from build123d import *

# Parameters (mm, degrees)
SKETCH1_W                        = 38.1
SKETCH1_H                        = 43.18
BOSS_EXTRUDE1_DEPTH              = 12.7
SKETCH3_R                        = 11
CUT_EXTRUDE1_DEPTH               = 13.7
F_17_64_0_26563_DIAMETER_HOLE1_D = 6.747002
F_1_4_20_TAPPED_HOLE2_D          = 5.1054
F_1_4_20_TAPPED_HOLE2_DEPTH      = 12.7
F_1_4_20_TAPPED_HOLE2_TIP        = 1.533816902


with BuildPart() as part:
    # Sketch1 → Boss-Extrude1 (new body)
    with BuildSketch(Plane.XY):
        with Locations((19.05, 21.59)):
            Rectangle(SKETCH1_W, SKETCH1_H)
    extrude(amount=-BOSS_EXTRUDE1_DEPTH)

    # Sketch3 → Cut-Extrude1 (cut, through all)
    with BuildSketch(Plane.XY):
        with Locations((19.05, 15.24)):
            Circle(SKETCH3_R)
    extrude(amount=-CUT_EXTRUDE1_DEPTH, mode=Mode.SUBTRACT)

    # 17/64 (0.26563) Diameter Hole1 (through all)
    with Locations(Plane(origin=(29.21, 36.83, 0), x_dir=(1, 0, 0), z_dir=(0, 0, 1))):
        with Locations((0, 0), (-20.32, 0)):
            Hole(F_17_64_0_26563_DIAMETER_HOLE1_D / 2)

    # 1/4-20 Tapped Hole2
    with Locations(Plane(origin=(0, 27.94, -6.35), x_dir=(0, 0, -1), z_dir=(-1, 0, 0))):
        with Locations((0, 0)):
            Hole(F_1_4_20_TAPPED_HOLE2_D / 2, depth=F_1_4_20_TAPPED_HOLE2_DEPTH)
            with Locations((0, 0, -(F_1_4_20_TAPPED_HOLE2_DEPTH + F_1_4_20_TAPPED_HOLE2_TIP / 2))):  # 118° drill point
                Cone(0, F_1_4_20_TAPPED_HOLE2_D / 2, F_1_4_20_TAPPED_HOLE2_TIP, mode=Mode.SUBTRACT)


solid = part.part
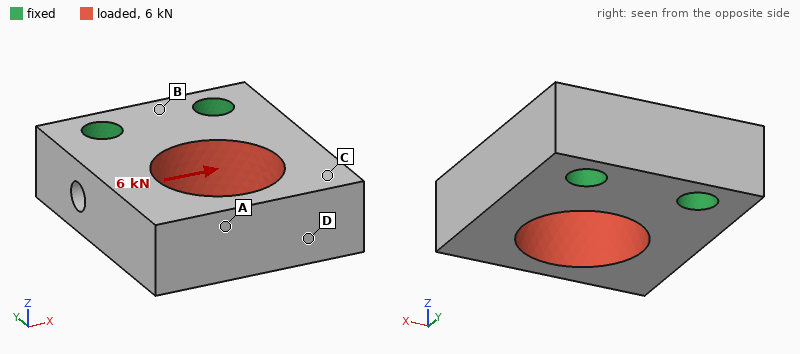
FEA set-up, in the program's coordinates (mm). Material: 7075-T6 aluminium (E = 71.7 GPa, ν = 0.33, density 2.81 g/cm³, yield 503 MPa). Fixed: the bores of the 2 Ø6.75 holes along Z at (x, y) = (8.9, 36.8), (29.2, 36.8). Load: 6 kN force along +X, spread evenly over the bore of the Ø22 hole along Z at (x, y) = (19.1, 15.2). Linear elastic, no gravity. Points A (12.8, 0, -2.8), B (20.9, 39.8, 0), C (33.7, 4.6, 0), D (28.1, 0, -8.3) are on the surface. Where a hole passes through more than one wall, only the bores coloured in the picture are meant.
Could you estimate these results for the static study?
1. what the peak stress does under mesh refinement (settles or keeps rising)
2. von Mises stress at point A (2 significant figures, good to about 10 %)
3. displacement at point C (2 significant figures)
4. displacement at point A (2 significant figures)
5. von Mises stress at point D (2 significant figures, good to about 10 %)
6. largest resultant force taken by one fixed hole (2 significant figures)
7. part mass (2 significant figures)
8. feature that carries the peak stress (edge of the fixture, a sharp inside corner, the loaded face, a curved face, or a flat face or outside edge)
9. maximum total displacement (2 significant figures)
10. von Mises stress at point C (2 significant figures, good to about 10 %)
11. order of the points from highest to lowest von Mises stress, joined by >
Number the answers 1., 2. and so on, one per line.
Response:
1. keeps rising
2. 62 MPa
3. 71 µm
4. 75 µm
5. 51 MPa
6. 5.1 kN
7. 42 g
8. a sharp inside corner
9. 83 µm
10. 23 MPa
11. A > D > C > B
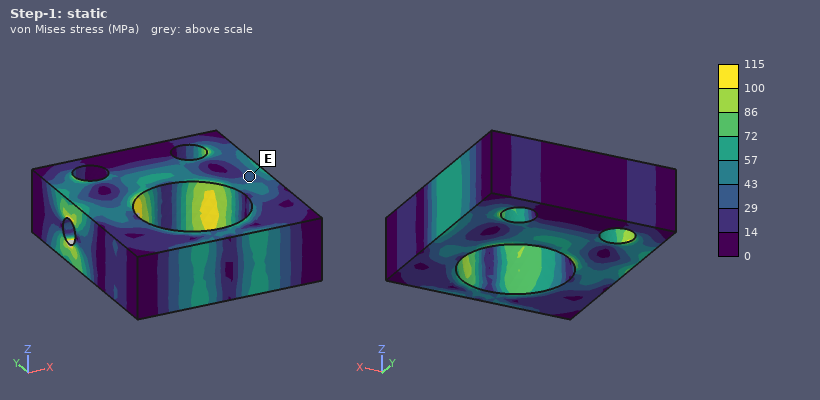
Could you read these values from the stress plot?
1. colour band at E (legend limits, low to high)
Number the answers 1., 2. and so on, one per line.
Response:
1. 29 to 43 MPa
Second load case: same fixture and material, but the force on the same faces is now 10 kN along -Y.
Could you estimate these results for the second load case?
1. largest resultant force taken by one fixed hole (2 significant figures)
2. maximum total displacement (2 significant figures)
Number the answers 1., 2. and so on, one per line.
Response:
1. 5.0 kN
2. 36 µm
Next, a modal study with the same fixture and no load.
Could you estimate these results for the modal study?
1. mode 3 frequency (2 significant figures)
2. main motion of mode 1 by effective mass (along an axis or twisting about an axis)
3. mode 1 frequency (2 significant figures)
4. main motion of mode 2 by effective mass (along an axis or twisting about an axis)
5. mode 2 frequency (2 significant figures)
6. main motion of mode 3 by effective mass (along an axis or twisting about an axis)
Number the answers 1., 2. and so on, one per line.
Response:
1. 11 kHz
2. along Z
3. 6900 Hz
4. along X
5. 9300 Hz
6. twisting about Y
